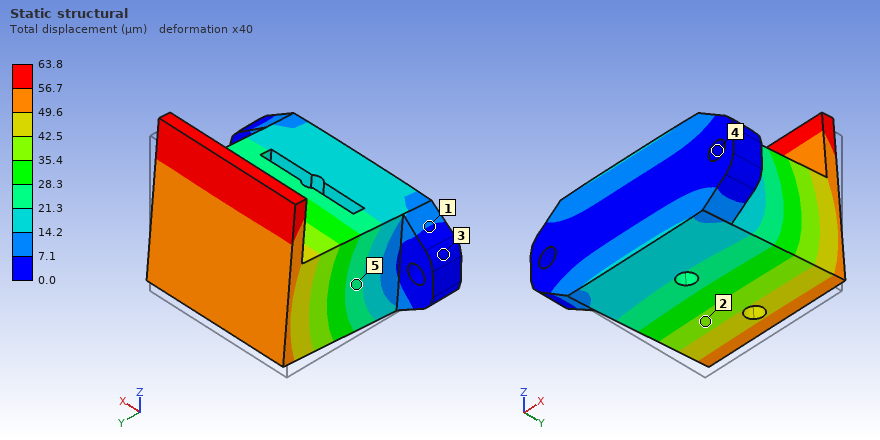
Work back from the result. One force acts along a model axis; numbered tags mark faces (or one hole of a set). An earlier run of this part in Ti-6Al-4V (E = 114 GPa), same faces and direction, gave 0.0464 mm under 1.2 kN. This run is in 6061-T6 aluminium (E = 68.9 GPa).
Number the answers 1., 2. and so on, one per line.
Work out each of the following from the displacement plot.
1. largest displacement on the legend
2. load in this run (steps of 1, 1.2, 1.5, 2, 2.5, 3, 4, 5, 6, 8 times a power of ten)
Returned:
1. 63.8 µm
2. 1 kN
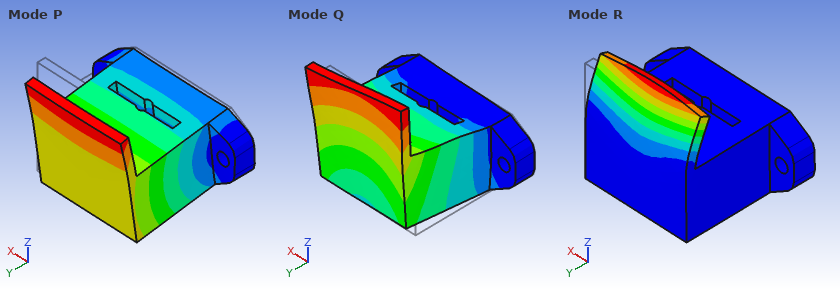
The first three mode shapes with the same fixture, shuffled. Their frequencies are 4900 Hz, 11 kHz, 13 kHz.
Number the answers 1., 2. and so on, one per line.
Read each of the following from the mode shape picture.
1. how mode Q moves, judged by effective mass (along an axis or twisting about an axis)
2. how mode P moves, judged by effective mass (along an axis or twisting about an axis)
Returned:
1. along X
2. along Z
